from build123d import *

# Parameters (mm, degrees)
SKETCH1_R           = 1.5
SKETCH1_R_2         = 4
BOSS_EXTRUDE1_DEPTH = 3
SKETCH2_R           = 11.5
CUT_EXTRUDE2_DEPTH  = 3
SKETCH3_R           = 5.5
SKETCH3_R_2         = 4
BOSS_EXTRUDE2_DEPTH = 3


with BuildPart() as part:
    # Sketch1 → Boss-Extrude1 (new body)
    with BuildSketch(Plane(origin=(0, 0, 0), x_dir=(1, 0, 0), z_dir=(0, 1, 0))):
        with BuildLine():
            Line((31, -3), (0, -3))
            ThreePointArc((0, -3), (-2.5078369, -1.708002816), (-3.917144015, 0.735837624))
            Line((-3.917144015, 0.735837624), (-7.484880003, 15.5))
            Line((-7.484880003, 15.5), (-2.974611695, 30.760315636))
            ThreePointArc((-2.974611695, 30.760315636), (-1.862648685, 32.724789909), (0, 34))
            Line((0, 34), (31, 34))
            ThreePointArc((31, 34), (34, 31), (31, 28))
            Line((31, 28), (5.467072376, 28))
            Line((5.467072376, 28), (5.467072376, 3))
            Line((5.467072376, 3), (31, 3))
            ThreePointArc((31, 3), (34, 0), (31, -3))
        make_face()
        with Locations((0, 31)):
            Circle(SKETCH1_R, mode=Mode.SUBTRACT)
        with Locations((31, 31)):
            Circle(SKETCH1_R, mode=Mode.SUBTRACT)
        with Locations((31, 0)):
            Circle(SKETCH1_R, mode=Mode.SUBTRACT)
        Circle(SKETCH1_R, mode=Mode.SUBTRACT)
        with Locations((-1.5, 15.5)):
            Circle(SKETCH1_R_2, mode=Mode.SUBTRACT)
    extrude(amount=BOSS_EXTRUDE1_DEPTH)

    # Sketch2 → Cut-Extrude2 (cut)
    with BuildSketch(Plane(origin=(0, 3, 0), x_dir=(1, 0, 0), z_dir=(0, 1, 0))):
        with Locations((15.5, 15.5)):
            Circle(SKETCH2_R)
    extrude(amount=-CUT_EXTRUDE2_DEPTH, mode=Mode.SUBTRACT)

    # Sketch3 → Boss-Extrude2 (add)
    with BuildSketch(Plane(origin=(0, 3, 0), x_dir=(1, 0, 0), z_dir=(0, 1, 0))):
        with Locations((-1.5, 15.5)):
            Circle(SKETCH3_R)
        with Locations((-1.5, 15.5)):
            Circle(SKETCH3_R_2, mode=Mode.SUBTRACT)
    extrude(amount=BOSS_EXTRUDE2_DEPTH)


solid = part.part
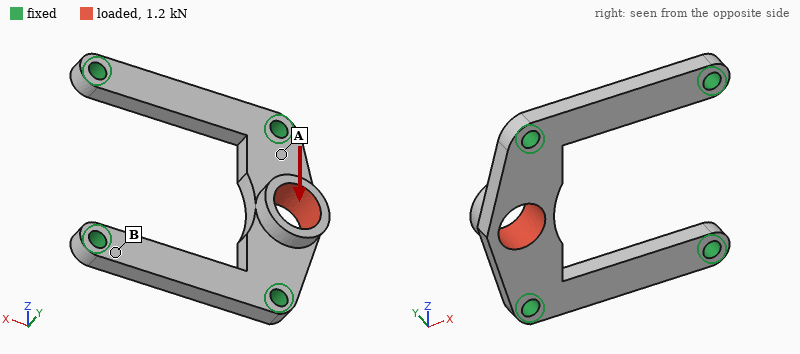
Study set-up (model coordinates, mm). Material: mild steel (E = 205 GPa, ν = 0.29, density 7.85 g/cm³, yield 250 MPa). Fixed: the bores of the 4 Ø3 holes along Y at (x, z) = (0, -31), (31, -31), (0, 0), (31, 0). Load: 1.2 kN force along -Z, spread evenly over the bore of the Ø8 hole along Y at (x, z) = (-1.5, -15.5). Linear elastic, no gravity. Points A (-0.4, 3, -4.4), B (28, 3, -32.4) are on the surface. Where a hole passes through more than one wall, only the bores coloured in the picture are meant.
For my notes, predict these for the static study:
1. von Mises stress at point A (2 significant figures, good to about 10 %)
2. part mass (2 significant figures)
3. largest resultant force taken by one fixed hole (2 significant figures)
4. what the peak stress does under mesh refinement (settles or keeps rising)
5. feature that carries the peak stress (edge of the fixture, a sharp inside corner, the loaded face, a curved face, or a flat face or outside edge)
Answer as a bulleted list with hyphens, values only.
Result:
- 28 MPa
- 16 g
- 610 N
- keeps rising
- edge of the fixture
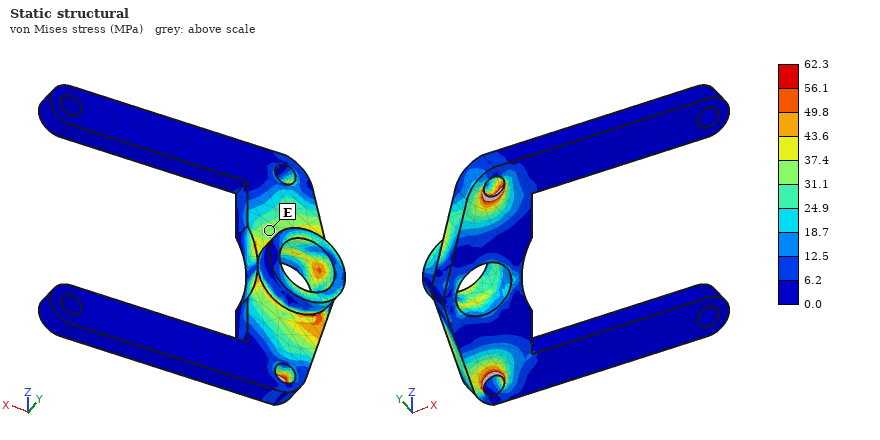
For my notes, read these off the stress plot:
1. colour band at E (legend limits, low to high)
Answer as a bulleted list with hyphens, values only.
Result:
- 31.1 to 37.4 MPa
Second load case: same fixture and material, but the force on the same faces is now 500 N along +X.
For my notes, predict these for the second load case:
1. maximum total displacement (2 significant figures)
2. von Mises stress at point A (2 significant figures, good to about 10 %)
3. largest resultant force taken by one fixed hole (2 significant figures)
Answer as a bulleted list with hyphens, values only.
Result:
- 8.5 µm
- 44 MPa
- 230 N
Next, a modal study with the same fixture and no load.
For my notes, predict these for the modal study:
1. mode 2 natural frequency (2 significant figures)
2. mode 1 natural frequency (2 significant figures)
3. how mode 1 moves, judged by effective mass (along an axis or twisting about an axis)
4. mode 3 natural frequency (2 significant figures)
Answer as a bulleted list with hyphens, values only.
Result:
- 18 kHz
- 16 kHz
- along Y
- 18 kHz
